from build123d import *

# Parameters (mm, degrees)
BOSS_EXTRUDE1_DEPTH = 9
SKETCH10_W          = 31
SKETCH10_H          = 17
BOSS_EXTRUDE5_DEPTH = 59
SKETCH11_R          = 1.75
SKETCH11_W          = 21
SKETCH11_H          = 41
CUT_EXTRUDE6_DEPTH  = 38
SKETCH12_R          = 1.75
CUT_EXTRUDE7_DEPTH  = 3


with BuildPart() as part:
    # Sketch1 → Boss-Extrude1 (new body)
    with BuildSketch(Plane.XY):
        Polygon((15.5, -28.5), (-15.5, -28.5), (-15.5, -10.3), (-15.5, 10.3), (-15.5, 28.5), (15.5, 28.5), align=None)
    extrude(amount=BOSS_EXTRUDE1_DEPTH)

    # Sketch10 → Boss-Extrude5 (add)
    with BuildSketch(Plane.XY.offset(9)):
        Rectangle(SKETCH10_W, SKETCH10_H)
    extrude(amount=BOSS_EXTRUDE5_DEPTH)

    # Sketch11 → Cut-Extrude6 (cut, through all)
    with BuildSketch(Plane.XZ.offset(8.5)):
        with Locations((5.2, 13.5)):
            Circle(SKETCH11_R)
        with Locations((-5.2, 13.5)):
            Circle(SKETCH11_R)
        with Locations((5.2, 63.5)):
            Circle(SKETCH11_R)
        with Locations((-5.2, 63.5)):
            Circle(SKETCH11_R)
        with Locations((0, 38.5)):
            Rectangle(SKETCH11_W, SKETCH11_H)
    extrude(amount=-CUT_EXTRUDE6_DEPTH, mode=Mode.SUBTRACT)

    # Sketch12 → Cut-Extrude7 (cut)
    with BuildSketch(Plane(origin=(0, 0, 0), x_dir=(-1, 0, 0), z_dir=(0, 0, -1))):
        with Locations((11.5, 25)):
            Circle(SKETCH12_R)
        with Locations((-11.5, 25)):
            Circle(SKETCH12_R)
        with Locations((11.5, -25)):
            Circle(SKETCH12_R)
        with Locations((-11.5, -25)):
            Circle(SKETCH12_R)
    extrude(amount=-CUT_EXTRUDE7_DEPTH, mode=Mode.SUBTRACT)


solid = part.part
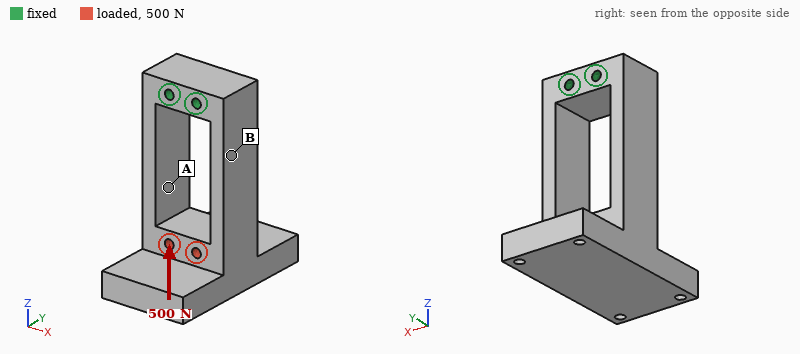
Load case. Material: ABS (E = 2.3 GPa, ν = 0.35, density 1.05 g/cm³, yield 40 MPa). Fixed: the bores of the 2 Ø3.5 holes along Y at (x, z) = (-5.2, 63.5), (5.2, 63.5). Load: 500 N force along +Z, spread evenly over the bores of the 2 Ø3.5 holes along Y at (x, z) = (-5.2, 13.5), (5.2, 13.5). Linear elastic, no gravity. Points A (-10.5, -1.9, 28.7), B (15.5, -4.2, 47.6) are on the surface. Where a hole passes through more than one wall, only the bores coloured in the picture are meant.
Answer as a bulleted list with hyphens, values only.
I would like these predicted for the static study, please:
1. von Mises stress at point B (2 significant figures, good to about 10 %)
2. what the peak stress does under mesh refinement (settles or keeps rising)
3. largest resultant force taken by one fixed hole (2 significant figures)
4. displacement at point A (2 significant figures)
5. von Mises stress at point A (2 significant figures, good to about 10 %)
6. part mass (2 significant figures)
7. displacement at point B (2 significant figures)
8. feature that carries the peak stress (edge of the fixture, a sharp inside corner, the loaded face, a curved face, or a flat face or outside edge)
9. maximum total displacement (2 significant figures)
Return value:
- 1.5 MPa
- keeps rising
- 250 N
- 0.089 mm
- 3.5 MPa
- 33 g
- 0.075 mm
- edge of the fixture
- 0.11 mm
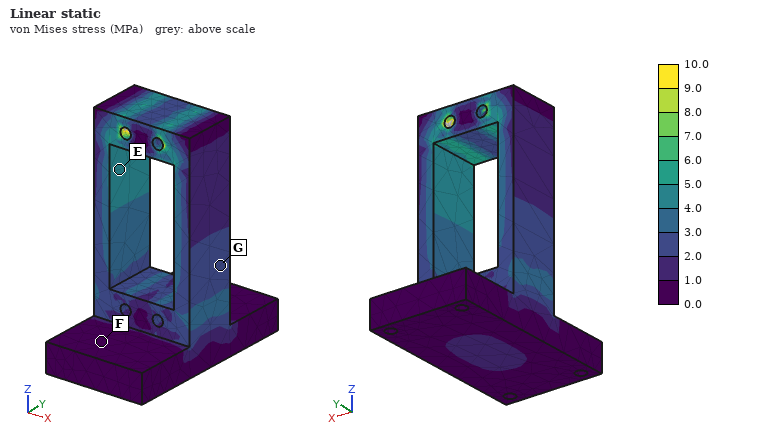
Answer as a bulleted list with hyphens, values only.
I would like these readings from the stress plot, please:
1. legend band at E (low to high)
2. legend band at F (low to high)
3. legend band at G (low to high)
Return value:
- 4.0 to 5.0 MPa
- 0.0 to 1.0 MPa
- 2.0 to 3.0 MPa
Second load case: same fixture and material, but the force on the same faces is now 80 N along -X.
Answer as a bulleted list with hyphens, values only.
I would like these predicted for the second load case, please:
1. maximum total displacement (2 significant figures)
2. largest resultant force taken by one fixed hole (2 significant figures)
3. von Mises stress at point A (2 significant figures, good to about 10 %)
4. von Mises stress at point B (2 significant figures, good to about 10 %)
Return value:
- 1.1 mm
- 190 N
- 6.3 MPa
- 5.8 MPa
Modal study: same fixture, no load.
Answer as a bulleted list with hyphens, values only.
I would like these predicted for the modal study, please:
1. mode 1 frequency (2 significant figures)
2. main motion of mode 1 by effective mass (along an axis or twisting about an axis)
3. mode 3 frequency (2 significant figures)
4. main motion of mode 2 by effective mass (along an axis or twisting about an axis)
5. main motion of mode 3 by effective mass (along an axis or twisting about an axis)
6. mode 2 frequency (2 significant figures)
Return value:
- 280 Hz
- along X
- 610 Hz
- along Y
- twisting about Z
- 320 Hz
